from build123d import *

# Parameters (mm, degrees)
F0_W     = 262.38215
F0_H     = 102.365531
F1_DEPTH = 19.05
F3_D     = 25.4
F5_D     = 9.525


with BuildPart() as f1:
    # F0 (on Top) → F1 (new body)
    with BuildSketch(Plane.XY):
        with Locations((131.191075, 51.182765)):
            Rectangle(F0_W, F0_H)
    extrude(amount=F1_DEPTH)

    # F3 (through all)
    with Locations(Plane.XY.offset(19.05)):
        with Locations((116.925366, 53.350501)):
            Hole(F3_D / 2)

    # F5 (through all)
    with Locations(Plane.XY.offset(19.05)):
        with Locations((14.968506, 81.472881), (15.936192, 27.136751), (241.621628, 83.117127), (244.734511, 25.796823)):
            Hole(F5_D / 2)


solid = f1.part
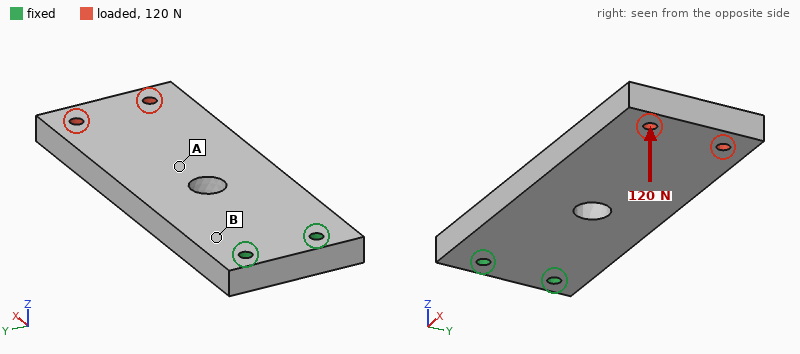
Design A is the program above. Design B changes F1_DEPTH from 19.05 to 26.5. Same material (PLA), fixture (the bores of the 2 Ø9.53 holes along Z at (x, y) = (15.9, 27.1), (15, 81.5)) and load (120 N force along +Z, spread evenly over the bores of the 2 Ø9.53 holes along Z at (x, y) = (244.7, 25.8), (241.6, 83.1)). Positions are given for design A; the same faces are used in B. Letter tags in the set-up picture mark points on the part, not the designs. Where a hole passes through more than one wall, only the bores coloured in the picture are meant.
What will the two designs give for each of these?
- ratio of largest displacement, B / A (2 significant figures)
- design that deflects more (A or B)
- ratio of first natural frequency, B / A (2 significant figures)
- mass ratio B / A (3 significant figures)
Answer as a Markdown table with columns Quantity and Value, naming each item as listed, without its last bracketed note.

| Quantity | Value |
|---|---|
| ratio of largest displacement, B / A | 0.38 |
| design that deflects more | A |
| ratio of first natural frequency, B / A | 1.4 |
| mass ratio B / A | 1.39 |
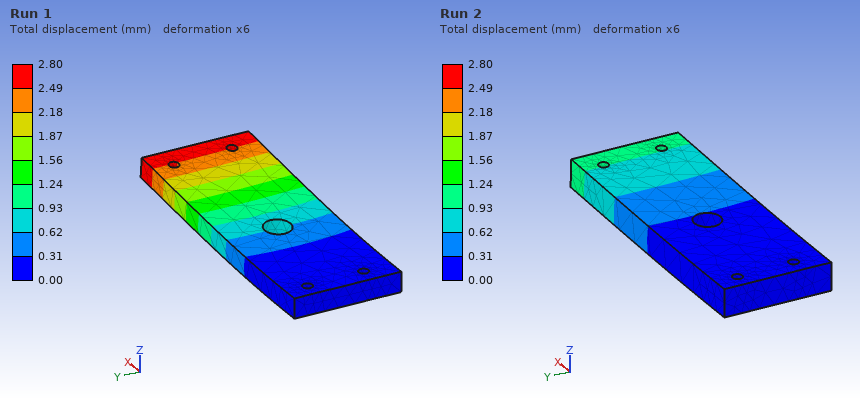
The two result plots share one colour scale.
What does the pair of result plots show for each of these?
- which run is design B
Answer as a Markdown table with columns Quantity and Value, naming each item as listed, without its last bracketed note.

| Quantity | Value |
|---|---|
| which run is design B | Run 2 |
